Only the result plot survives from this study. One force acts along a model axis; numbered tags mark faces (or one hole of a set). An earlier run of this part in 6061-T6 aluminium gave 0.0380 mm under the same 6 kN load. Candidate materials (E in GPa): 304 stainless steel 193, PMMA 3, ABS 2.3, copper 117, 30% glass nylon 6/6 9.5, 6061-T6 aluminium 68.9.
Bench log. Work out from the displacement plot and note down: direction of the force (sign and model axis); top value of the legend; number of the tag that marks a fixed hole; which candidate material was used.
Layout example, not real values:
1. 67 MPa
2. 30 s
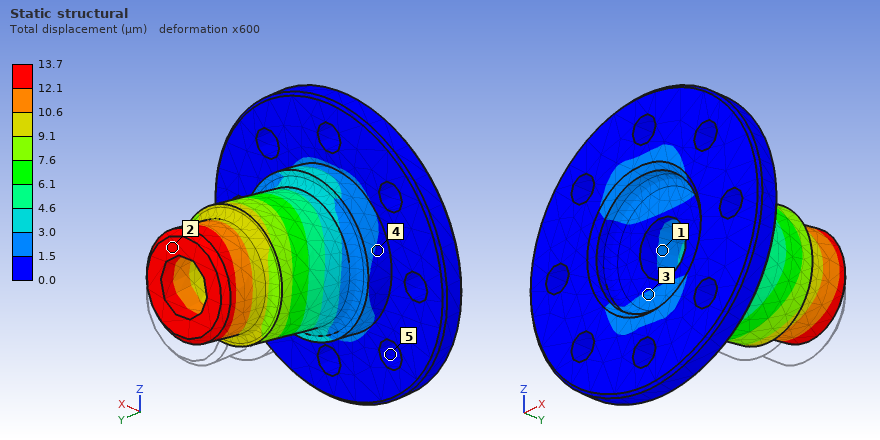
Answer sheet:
1. +Z
2. 13.7 µm
3. 5
4. 304 stainless steel
